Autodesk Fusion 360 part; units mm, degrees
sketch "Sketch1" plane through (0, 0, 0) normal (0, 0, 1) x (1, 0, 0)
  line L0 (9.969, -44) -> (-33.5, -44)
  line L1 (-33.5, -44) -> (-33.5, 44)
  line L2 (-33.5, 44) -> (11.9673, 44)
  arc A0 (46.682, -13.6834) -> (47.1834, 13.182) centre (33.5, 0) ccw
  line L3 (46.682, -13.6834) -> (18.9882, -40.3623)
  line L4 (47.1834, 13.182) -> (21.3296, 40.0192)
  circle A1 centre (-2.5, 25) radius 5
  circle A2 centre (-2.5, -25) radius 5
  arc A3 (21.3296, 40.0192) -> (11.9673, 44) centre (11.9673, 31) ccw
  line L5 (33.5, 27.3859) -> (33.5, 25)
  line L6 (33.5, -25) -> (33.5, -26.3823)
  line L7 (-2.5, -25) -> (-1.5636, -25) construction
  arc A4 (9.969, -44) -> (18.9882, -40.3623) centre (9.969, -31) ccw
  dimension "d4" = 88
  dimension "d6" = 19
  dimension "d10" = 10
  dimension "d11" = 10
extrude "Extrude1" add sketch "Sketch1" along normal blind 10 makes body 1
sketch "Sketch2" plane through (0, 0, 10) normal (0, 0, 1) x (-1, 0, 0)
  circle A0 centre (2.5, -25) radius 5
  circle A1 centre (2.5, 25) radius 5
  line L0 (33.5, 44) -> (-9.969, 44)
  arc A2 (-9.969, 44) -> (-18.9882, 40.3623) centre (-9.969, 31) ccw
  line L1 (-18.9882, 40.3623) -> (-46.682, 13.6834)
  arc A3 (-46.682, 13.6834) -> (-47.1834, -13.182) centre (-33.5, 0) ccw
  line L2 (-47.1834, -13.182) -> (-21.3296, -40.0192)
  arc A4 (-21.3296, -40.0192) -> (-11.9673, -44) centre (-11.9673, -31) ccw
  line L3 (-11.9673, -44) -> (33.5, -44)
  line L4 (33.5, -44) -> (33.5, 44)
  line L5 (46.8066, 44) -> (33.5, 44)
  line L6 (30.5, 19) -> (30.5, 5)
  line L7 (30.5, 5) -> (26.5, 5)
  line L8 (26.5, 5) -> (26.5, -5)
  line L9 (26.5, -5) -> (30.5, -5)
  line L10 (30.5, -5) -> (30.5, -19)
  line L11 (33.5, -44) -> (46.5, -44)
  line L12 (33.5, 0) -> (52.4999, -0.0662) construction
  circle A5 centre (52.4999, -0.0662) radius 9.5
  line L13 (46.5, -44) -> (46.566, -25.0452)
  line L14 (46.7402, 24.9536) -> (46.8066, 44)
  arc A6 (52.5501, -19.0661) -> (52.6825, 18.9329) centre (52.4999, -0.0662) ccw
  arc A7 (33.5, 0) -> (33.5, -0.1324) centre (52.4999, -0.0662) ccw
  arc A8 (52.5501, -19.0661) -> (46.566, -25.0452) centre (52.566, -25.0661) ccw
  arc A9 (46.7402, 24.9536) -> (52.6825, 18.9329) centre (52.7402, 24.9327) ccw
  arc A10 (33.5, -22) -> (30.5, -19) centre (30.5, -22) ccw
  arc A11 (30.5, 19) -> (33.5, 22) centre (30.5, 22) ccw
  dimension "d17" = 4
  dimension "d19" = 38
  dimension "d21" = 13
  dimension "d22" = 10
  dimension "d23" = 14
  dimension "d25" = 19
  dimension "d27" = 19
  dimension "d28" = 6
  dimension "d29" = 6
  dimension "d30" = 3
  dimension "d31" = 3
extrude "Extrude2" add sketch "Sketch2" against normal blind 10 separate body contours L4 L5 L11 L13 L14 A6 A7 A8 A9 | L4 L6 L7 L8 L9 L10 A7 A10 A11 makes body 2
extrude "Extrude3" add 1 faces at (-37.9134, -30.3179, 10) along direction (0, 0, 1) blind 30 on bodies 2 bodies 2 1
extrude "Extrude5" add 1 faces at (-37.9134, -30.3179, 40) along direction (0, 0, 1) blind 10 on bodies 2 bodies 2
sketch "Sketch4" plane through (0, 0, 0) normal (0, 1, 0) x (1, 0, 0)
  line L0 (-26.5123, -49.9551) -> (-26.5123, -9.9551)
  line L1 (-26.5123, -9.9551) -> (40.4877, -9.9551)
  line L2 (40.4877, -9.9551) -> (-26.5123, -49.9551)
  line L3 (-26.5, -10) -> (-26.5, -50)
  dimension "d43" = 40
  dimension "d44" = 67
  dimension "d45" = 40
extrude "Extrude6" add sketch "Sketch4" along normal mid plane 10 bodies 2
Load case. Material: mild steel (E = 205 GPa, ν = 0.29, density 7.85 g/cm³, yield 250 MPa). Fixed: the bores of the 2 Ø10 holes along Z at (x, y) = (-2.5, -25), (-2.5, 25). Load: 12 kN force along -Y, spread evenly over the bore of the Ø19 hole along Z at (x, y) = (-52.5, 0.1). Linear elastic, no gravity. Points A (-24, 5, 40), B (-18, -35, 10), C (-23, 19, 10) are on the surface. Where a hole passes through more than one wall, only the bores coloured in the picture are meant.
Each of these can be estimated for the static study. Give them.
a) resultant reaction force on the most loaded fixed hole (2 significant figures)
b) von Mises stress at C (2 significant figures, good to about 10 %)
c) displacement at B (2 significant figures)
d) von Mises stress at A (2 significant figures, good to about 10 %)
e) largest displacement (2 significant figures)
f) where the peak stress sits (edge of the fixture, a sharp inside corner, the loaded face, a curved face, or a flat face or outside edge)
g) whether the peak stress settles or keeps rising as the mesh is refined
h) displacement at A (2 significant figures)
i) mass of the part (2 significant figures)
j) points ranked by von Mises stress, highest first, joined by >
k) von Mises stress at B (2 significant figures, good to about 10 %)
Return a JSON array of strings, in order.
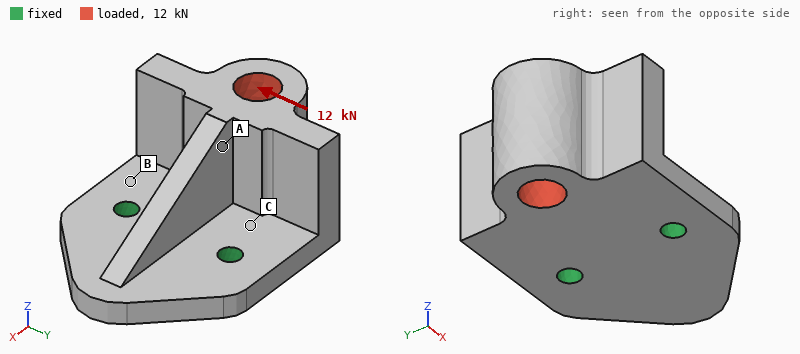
["13 kN", "71 MPa", "12 µm", "18 MPa", "56 µm", "edge of the fixture", "keeps rising", "32 µm", "1.3 kg", "C > B > A", "37 MPa"]
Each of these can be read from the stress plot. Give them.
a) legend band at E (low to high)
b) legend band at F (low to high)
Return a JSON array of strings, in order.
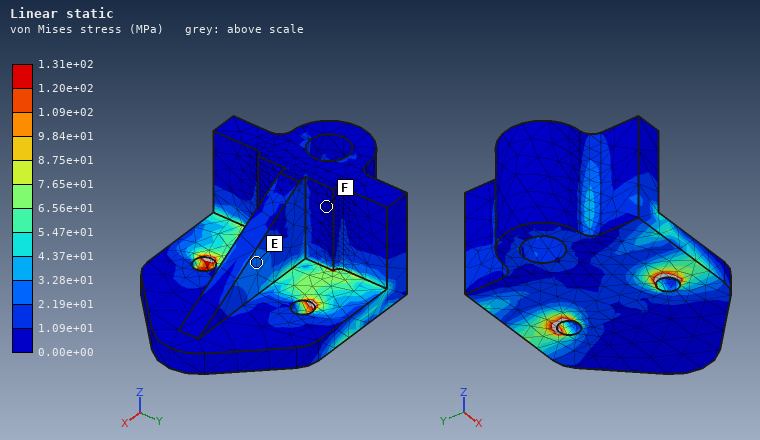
["2.19e+01 to 3.28e+01 MPa", "0.00e+00 to 1.09e+01 MPa"]
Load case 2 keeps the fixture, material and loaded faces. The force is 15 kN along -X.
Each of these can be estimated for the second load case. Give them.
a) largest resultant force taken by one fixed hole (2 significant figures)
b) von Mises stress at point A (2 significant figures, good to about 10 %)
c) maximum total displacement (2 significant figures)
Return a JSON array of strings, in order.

["7.5 kN", "37 MPa", "0.14 mm"]
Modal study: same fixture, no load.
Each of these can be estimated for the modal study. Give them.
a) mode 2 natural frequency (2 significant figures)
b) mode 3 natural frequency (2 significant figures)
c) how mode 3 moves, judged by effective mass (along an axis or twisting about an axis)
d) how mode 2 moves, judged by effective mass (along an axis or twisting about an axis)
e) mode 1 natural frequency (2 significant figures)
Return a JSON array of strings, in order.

["2900 Hz", "5500 Hz", "along Z", "along Y", "1600 Hz"]
